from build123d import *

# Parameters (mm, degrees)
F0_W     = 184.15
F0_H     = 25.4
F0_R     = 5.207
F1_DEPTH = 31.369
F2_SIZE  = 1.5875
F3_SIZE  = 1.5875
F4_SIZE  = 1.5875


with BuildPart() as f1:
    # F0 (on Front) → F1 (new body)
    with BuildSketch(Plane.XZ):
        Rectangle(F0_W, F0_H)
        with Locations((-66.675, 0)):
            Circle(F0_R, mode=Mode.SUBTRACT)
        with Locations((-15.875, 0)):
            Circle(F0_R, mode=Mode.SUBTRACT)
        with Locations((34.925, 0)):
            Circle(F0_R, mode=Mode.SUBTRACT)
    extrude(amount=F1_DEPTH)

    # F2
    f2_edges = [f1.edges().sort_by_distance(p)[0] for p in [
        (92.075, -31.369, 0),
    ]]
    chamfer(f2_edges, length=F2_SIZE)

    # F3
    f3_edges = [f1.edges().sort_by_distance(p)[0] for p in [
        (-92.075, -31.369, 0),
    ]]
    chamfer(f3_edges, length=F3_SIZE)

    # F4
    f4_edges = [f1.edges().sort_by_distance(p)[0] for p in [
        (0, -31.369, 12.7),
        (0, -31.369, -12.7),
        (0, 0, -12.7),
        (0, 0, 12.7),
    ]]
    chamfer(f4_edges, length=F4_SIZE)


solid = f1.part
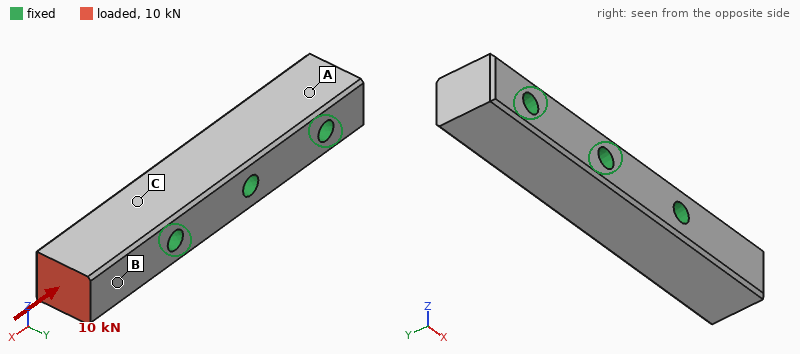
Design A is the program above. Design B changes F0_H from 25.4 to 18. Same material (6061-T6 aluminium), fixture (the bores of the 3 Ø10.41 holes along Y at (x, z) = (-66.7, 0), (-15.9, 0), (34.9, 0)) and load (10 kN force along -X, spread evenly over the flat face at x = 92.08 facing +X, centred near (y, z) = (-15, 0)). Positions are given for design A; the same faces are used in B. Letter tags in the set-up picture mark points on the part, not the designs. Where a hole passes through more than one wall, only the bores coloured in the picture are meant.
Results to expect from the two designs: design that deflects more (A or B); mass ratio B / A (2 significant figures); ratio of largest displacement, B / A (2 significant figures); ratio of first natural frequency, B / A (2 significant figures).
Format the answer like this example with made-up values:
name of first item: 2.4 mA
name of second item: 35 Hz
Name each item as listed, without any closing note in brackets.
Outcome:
design that deflects more: B
mass ratio B / A: 0.69
ratio of largest displacement, B / A: 1.4
ratio of first natural frequency, B / A: 0.85
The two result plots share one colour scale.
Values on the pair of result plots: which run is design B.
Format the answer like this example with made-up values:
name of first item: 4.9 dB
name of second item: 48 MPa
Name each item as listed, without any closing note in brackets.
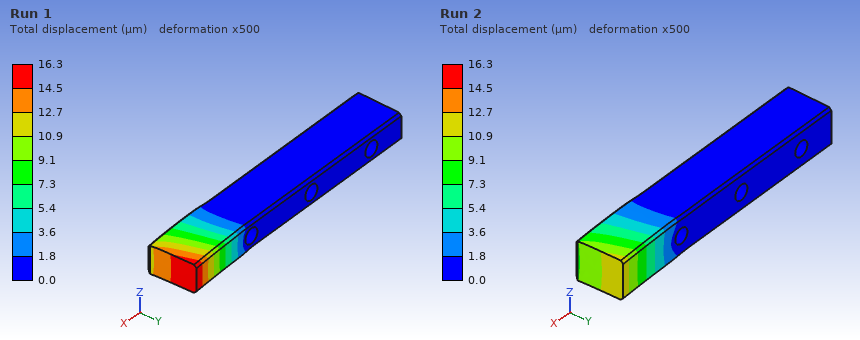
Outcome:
which run is design B: Run 1
